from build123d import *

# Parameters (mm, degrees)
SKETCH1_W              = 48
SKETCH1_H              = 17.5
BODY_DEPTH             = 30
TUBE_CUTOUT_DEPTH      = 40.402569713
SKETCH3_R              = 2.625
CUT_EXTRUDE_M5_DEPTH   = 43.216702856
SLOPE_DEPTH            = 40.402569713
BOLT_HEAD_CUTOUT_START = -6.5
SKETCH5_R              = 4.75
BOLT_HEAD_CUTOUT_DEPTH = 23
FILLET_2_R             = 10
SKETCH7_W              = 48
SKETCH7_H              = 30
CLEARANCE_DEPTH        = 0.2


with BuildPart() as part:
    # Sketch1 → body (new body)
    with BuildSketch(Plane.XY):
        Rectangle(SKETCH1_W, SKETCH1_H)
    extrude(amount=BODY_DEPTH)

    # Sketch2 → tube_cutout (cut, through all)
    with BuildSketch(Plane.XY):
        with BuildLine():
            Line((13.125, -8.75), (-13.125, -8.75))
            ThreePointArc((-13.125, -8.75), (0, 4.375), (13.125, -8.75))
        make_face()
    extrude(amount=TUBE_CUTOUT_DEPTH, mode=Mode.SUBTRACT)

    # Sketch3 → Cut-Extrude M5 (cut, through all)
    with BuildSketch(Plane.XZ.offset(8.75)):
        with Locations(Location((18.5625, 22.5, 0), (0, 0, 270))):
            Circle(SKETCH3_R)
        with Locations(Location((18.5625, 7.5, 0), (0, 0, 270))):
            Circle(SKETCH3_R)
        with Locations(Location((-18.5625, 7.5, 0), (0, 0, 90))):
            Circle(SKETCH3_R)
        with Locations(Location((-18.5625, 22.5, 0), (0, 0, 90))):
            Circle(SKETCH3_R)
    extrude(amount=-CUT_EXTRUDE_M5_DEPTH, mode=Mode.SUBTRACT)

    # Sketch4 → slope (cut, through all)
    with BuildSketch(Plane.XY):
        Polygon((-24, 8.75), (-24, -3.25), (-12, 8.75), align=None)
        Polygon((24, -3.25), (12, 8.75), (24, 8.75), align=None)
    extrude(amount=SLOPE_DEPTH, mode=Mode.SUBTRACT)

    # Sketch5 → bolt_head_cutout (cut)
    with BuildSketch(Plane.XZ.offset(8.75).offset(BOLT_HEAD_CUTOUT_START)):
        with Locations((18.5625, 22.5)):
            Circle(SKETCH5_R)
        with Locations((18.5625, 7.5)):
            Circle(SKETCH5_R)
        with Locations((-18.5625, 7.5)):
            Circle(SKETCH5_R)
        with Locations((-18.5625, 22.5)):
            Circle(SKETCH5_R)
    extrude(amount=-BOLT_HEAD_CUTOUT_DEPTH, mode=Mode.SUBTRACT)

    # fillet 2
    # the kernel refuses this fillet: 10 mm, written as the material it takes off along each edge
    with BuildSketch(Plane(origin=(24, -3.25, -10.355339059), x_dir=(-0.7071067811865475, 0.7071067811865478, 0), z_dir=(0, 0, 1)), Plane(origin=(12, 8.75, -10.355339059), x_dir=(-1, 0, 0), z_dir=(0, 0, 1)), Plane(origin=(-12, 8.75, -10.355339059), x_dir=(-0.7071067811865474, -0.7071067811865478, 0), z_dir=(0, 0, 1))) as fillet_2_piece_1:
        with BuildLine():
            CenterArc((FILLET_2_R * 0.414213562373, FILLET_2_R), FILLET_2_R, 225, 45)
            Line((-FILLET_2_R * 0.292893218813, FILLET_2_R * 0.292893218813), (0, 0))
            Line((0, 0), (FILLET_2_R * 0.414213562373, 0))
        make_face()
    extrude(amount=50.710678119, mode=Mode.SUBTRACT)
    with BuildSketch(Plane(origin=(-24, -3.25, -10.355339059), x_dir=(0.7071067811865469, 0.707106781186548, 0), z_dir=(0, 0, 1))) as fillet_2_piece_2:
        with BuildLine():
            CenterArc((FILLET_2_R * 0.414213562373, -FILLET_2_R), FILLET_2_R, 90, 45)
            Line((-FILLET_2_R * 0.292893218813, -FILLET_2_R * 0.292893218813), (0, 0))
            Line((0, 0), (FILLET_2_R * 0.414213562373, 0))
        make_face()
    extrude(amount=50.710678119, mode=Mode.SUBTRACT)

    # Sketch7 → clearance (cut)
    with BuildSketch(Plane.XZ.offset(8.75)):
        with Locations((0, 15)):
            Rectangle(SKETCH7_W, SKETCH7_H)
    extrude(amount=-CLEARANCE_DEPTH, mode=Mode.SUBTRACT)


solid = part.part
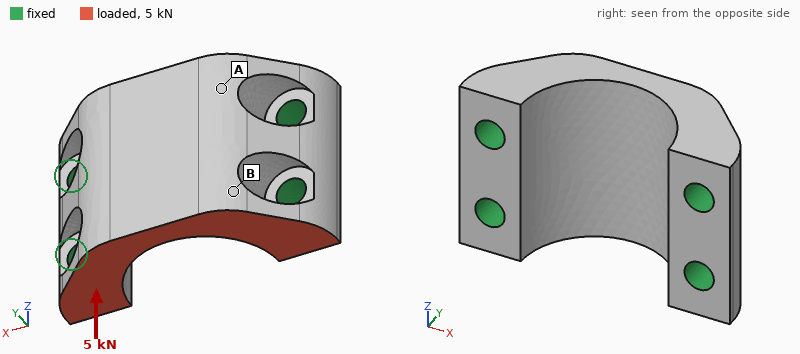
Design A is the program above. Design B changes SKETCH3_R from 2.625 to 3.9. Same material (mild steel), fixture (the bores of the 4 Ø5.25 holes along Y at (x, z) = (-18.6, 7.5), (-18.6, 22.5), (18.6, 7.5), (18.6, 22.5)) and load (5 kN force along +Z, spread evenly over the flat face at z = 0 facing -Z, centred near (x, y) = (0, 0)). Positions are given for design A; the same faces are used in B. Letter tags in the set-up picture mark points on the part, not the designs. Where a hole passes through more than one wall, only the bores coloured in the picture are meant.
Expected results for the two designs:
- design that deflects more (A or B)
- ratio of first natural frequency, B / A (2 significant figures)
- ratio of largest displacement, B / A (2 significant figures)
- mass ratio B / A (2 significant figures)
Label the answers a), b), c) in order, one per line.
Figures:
a) A
b) 1.2
c) 0.79
d) 0.94
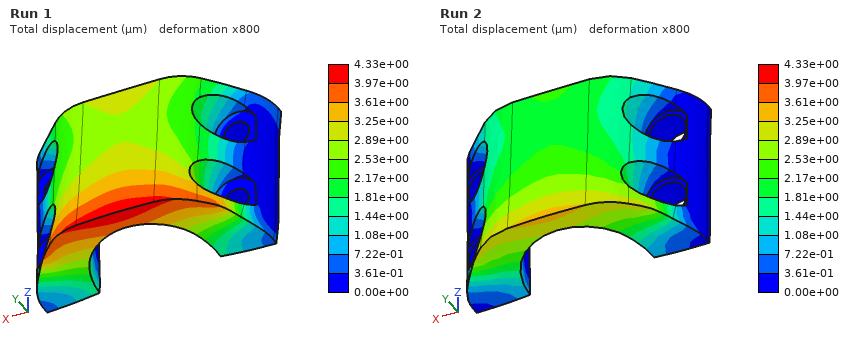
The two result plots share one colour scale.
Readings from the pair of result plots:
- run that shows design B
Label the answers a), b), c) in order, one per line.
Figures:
a) Run 2
